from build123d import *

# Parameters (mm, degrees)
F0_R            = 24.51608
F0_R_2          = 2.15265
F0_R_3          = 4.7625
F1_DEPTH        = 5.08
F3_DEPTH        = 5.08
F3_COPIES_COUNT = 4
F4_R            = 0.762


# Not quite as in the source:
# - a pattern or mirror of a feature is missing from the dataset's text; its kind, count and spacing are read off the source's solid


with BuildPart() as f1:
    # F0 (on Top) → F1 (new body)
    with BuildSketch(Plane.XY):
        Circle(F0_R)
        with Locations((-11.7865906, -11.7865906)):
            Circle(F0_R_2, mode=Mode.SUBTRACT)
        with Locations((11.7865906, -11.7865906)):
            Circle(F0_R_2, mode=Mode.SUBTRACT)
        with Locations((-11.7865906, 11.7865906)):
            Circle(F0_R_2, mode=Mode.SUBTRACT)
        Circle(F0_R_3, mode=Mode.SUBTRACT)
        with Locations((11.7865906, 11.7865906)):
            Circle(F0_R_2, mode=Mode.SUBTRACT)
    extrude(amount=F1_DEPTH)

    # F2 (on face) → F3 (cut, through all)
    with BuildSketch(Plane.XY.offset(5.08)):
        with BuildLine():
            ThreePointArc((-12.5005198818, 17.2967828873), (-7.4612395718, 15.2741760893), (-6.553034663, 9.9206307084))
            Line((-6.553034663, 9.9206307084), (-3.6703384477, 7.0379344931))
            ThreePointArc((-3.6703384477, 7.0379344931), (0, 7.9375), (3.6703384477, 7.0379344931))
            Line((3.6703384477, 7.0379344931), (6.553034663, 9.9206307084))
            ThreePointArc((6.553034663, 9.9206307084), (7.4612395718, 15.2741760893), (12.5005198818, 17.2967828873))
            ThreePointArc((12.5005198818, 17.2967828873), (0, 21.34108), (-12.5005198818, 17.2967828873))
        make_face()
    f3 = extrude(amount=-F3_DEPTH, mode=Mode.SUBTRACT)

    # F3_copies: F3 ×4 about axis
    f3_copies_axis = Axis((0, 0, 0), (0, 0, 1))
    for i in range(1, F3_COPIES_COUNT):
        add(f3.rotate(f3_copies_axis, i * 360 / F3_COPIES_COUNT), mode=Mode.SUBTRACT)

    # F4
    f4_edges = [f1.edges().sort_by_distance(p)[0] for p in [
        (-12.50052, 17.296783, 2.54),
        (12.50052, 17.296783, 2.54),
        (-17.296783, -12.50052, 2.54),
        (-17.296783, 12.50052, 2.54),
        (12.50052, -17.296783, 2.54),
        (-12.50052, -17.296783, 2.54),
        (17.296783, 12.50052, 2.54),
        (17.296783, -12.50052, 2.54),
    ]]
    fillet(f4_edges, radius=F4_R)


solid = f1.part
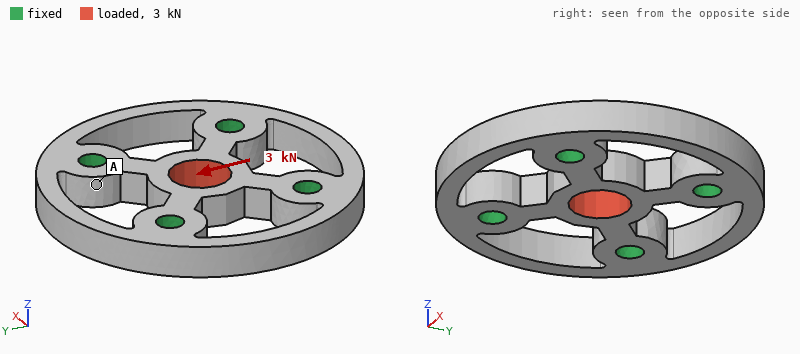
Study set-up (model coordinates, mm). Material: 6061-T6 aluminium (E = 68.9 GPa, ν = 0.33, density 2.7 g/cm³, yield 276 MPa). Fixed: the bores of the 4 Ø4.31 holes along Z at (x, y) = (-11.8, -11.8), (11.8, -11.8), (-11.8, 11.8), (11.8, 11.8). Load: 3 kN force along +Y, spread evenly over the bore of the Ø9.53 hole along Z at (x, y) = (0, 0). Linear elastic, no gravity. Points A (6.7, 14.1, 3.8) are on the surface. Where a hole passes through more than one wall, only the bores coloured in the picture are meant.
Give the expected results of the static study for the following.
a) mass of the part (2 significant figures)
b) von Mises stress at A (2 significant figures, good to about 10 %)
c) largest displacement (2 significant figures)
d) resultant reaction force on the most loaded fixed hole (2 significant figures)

13 g
7.8 MPa
13 µm
890 N
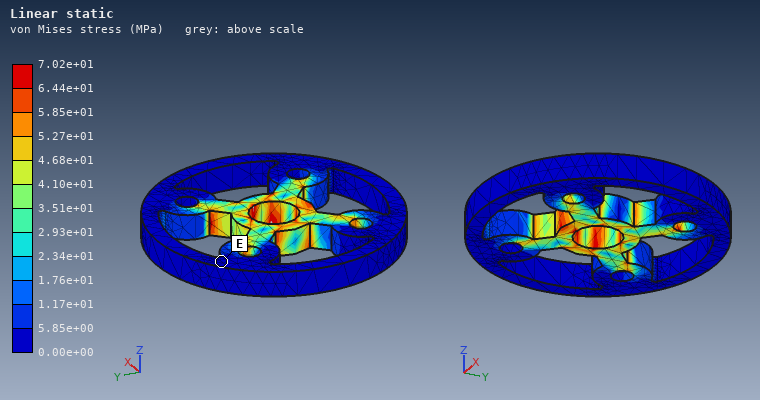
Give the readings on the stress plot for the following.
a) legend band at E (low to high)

0.00e+00 to 5.85e+00 MPa
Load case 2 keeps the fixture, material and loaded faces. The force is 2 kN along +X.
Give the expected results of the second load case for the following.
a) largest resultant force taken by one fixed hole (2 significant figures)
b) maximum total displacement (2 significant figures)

590 N
8.7 µm
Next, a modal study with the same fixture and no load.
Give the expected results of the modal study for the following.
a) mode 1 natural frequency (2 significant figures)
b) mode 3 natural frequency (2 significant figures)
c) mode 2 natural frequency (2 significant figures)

17 kHz
19 kHz
19 kHz
